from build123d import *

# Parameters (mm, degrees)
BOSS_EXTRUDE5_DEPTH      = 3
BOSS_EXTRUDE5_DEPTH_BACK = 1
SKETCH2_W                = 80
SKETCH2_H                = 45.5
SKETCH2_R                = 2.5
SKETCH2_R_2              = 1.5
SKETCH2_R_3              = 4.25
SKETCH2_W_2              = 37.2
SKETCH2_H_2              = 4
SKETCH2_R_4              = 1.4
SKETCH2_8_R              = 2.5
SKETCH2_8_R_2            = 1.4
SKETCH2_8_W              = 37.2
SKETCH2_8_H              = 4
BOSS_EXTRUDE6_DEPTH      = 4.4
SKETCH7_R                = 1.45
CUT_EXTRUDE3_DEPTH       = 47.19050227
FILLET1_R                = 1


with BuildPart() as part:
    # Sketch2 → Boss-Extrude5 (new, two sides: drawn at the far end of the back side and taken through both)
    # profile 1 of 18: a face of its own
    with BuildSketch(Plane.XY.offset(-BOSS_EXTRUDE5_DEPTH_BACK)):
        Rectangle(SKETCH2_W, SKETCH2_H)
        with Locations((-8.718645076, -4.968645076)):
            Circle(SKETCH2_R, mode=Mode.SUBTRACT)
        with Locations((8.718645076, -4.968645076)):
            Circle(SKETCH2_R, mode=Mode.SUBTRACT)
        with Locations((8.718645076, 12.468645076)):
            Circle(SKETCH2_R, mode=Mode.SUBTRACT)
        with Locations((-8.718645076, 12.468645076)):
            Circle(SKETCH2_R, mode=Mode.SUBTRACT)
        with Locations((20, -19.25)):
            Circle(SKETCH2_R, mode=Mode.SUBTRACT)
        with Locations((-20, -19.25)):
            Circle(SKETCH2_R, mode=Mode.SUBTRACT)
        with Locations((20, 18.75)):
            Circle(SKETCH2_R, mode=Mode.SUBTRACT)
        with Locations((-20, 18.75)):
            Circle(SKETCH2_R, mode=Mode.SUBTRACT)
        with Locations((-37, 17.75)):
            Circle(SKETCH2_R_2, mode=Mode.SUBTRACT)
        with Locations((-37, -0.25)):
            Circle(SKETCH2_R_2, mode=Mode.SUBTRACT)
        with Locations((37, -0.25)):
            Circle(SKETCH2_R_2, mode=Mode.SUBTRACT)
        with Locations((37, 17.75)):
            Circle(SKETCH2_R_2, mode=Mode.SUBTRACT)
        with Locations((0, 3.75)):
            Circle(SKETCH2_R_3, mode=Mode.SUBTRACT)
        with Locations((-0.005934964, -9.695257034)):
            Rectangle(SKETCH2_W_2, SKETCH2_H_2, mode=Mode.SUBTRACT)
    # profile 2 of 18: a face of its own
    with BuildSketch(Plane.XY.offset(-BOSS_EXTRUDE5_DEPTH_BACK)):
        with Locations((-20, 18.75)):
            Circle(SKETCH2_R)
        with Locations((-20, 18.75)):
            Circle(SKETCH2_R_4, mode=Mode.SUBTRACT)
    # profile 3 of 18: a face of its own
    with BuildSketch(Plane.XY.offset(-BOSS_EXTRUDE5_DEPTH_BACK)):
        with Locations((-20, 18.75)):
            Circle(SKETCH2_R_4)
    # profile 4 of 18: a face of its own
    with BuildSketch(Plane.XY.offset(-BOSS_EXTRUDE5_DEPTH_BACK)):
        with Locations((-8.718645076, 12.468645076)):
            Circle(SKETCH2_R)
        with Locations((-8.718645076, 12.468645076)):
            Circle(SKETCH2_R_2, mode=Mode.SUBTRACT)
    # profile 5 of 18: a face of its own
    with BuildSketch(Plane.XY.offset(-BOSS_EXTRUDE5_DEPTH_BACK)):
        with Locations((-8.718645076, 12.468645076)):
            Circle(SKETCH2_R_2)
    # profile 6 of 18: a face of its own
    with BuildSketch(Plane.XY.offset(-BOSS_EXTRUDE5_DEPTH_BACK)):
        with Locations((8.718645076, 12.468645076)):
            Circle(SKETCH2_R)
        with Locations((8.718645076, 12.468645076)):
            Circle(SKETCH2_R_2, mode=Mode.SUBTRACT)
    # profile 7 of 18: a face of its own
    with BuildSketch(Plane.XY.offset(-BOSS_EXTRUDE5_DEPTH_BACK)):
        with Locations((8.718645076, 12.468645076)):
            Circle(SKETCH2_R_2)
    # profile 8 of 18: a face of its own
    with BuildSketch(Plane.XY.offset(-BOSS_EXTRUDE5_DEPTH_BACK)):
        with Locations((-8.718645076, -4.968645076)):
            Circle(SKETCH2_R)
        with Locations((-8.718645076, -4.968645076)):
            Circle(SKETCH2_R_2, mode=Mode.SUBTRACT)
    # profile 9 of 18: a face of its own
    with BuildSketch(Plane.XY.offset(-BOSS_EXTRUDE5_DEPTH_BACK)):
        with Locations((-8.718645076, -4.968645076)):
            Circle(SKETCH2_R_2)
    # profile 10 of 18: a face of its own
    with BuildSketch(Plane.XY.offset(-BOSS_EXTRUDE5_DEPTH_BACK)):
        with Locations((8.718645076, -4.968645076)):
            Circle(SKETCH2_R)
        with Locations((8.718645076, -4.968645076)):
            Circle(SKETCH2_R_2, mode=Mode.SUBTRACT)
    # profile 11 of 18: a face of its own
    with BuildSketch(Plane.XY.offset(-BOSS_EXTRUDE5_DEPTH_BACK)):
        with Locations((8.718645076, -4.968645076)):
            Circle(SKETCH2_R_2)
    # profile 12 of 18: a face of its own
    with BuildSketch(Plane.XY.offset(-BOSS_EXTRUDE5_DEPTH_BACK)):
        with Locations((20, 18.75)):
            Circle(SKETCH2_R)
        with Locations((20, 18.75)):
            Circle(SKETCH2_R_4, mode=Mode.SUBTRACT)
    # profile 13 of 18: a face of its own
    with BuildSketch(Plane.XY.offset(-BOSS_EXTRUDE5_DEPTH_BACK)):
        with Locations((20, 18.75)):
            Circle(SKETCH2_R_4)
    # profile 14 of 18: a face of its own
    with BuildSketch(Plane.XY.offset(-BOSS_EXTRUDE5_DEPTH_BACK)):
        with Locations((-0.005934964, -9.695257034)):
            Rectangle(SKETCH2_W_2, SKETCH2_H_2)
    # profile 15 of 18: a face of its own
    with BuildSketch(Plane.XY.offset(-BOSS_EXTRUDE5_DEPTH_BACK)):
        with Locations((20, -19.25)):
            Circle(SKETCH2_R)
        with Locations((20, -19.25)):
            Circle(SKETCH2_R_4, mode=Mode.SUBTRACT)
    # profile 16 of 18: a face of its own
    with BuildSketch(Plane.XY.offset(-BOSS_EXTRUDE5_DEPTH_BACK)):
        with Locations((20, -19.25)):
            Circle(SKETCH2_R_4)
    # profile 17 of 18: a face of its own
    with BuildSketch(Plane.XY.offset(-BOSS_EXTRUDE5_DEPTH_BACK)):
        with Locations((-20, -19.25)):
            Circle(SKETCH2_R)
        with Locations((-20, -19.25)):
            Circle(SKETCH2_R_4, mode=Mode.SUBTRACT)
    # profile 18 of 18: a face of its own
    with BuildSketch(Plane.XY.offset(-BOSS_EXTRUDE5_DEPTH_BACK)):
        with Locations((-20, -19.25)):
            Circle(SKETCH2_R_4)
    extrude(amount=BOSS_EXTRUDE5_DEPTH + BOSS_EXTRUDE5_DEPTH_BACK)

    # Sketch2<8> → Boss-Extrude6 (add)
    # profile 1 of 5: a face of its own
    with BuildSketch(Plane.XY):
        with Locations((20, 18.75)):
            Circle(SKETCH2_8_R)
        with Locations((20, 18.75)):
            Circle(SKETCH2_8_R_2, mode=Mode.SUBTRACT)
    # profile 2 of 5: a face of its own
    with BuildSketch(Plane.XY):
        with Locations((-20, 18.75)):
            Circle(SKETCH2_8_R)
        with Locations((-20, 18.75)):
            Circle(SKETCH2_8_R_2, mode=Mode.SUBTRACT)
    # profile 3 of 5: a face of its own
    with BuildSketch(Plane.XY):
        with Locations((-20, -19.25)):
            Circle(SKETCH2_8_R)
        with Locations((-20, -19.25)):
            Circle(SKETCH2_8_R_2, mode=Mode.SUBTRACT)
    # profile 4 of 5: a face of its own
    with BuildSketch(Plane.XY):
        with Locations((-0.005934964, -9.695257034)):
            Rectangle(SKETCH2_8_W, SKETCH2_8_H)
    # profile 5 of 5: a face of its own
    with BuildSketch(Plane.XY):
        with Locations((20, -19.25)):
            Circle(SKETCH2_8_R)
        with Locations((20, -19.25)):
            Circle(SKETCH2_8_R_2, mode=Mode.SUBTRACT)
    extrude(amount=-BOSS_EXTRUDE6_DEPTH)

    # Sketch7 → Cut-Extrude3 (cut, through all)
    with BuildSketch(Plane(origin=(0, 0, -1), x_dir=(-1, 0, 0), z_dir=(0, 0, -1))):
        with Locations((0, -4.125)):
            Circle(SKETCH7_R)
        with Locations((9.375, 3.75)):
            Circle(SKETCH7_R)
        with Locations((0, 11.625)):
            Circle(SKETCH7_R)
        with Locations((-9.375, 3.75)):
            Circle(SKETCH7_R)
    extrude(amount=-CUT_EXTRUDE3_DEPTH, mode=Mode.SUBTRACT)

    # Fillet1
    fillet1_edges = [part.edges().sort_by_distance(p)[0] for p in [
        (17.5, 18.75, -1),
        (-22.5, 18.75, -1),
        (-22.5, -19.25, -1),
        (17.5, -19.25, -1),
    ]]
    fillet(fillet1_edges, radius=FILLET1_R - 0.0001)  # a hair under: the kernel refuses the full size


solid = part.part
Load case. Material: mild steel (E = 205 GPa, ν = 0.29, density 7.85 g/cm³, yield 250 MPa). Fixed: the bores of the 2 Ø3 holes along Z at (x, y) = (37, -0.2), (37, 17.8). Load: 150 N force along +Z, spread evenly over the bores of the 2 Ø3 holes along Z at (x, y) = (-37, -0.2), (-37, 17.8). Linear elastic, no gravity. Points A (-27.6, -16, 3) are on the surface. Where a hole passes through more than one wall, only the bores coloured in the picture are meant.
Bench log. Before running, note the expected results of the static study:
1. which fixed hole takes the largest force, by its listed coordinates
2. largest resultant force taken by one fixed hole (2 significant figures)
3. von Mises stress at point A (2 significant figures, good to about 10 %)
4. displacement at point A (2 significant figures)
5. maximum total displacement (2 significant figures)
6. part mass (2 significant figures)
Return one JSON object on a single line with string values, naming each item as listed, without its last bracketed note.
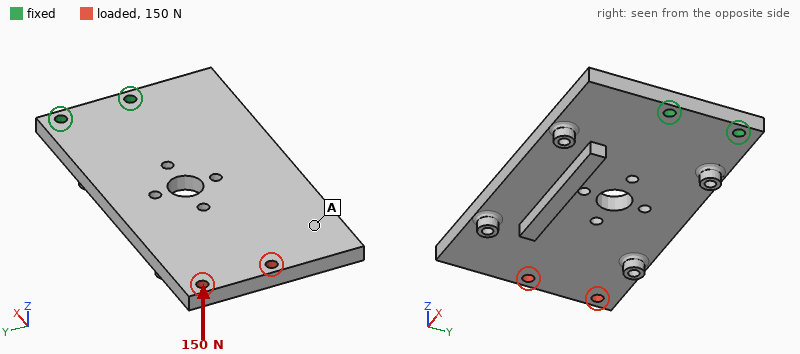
{"which fixed hole takes the largest force, by its listed coordinates": "(37, -0.2)", "largest resultant force taken by one fixed hole": "110 N", "von Mises stress at point A": "18 MPa", "displacement at point A": "0.34 mm", "maximum total displacement": "0.47 mm", "part mass": "120 g"}
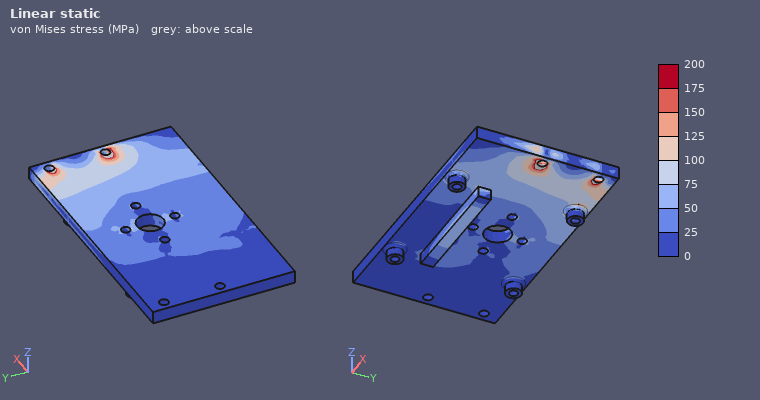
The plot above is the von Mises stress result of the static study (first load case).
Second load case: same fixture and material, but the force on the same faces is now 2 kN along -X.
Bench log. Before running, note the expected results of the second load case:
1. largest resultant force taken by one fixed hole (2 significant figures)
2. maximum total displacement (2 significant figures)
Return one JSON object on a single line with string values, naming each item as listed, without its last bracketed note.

{"largest resultant force taken by one fixed hole": "1.0 kN", "maximum total displacement": "12 µm"}
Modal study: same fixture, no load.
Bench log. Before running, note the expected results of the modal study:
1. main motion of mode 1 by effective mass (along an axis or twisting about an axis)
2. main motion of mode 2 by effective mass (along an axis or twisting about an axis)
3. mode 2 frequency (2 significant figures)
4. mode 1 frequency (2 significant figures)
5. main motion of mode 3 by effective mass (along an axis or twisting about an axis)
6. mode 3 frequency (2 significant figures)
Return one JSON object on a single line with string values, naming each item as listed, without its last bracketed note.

{"main motion of mode 1 by effective mass": "along Z", "main motion of mode 2 by effective mass": "twisting about X", "mode 2 frequency": "1800 Hz", "mode 1 frequency": "520 Hz", "main motion of mode 3 by effective mass": "along Y", "mode 3 frequency": "3000 Hz"}
